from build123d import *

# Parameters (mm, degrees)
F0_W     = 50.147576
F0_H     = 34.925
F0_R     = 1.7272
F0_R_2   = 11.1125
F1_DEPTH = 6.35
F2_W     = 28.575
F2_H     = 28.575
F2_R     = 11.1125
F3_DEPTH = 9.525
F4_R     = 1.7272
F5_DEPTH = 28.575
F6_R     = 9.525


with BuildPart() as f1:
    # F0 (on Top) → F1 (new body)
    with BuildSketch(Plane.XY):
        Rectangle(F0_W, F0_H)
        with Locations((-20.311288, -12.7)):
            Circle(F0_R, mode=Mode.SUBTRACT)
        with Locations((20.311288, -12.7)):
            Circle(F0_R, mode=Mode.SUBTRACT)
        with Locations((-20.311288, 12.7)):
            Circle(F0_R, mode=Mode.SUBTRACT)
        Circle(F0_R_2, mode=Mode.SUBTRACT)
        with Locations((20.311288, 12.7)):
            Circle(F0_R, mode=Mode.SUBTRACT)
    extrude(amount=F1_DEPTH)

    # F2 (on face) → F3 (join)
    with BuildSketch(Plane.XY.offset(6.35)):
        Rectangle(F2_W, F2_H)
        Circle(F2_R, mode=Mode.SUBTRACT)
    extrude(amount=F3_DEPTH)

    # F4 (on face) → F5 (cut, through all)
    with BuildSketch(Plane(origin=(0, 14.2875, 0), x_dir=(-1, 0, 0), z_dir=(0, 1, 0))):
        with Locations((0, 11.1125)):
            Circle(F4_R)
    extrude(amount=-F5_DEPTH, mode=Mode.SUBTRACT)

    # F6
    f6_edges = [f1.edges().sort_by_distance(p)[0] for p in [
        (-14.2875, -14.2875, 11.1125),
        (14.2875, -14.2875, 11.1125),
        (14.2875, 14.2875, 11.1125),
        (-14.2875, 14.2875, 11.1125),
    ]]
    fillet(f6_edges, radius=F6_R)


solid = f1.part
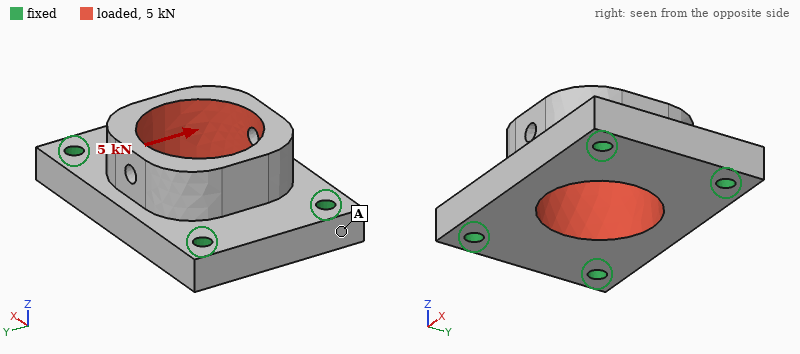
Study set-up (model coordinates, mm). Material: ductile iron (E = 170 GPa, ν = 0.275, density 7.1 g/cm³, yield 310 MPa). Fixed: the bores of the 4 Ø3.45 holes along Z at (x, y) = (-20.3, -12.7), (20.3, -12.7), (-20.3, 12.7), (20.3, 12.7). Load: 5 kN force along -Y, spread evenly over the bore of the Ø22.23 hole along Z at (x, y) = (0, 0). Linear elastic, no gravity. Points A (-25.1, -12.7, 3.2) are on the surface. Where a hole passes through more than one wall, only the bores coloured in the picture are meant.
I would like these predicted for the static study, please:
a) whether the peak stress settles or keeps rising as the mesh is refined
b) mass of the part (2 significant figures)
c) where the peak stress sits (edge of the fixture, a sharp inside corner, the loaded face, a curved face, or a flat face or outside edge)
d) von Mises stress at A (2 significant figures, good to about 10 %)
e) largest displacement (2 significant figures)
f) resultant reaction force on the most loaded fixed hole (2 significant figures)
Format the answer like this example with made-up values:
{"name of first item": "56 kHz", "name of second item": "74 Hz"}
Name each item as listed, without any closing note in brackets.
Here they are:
{"whether the peak stress settles or keeps rising as the mesh is refined": "keeps rising", "mass of the part": "83 g", "where the peak stress sits": "edge of the fixture", "von Mises stress at A": "9.8 MPa", "largest displacement": "9.1 µm", "resultant reaction force on the most loaded fixed hole": "1.5 kN"}
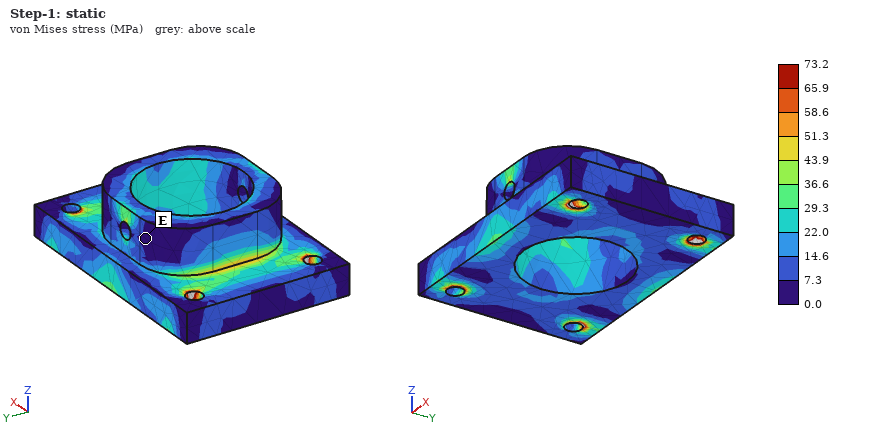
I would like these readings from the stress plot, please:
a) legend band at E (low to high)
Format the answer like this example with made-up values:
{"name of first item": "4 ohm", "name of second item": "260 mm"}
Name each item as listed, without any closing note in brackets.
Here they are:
{"legend band at E": "0.0 to 7.3 MPa"}
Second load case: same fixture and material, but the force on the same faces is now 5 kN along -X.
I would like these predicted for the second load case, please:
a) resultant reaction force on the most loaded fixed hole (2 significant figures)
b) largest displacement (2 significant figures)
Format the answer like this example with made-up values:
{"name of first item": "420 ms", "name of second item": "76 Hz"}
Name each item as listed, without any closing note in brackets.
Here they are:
{"resultant reaction force on the most loaded fixed hole": "1.3 kN", "largest displacement": "5.2 µm"}
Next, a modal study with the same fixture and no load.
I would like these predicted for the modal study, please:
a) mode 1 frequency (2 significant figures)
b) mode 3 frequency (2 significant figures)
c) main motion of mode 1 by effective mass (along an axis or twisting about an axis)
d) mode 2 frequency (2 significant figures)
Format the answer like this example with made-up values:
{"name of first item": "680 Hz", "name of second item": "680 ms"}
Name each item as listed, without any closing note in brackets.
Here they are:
{"mode 1 frequency": "17 kHz", "mode 3 frequency": "26 kHz", "main motion of mode 1 by effective mass": "along Z", "mode 2 frequency": "18 kHz"}
